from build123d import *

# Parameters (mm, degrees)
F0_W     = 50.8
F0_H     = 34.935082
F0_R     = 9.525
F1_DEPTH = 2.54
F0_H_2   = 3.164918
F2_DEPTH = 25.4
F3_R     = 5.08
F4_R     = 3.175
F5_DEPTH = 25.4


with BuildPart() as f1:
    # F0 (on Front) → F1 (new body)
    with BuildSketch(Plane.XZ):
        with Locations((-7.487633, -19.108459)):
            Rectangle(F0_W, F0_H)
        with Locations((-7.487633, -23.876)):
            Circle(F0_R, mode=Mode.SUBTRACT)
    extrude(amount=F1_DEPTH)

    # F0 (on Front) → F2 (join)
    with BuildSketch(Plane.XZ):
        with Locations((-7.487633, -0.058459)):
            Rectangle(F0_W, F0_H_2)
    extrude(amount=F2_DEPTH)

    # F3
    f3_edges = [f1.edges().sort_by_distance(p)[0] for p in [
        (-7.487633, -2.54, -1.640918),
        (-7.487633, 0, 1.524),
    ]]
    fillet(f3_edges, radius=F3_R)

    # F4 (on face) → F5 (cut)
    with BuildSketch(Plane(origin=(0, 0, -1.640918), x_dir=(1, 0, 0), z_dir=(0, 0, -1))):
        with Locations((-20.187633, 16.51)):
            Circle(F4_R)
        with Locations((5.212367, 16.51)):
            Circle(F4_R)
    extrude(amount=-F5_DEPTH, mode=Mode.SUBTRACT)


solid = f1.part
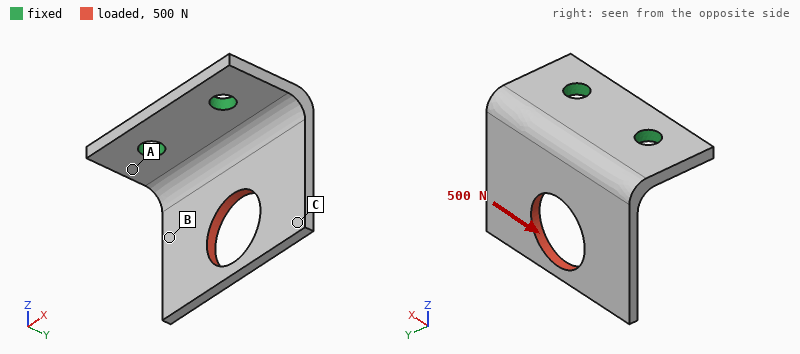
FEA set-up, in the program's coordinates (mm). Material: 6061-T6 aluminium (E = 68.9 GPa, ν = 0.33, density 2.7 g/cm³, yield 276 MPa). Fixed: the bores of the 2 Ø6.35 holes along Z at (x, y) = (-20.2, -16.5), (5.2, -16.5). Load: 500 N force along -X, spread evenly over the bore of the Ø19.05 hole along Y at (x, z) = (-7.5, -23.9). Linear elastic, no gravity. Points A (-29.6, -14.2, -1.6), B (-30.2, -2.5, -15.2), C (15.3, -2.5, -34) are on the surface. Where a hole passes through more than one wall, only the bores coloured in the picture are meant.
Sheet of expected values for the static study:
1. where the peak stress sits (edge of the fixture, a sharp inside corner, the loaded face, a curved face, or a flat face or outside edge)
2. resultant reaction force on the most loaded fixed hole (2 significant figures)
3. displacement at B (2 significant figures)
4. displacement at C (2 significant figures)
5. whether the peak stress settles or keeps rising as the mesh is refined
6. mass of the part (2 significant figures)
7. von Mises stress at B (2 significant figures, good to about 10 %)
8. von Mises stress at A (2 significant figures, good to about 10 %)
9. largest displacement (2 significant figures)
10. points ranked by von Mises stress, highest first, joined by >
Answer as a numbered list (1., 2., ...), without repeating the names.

1. edge of the fixture
2. 520 N
3. 0.098 mm
4. 0.16 mm
5. keeps rising
6. 21 g
7. 23 MPa
8. 44 MPa
9. 0.17 mm
10. A > B > C
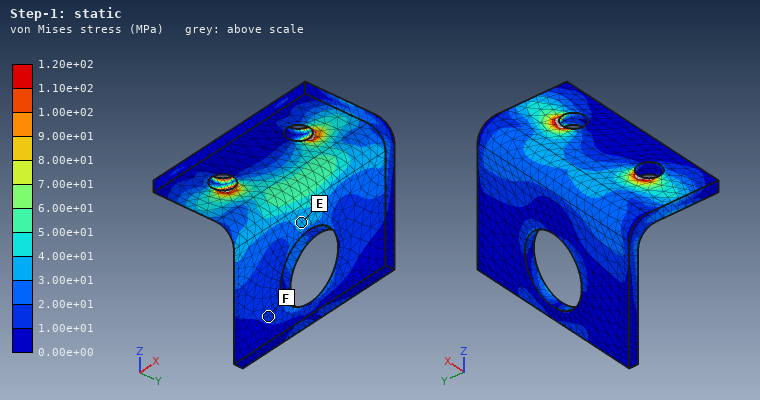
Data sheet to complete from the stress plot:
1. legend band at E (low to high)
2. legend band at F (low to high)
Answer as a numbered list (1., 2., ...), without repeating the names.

1. 3.00e+01 to 4.00e+01 MPa
2. 1.00e+01 to 2.00e+01 MPa
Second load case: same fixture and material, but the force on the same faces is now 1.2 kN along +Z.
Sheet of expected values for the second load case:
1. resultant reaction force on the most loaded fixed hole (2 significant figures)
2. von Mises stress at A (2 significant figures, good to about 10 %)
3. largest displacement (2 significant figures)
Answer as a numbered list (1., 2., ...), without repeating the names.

1. 600 N
2. 84 MPa
3. 0.46 mm
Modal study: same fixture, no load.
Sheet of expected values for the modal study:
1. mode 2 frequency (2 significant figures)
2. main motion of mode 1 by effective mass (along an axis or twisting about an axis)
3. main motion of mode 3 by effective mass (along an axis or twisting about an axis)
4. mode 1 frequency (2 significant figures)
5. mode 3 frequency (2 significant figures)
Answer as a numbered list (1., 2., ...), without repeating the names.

1. 2500 Hz
2. along Y
3. along X
4. 1500 Hz
5. 4100 Hz
